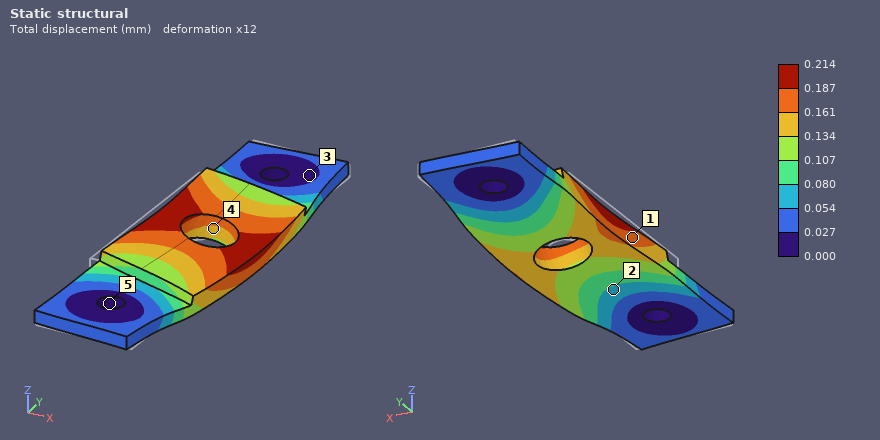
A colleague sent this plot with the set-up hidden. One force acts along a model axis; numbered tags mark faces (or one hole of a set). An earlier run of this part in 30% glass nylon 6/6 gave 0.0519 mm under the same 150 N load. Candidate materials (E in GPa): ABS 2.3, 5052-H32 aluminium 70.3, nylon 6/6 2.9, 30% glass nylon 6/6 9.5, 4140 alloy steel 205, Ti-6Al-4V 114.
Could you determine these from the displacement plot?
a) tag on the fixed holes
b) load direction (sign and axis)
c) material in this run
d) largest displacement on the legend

5
+X
ABS
0.214 mm
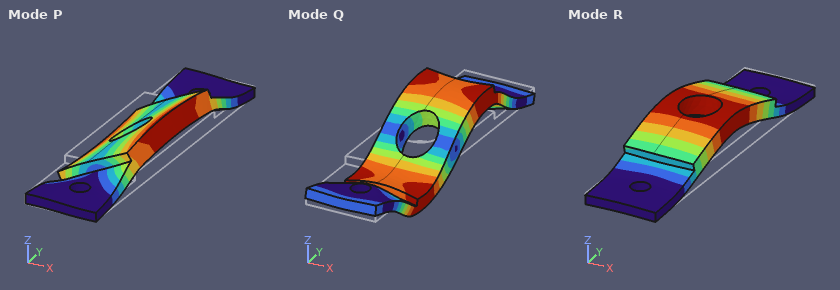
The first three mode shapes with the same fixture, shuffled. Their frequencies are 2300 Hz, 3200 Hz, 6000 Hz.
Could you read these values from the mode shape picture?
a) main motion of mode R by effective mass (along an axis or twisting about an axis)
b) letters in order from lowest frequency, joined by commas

along Z
R, P, Q
